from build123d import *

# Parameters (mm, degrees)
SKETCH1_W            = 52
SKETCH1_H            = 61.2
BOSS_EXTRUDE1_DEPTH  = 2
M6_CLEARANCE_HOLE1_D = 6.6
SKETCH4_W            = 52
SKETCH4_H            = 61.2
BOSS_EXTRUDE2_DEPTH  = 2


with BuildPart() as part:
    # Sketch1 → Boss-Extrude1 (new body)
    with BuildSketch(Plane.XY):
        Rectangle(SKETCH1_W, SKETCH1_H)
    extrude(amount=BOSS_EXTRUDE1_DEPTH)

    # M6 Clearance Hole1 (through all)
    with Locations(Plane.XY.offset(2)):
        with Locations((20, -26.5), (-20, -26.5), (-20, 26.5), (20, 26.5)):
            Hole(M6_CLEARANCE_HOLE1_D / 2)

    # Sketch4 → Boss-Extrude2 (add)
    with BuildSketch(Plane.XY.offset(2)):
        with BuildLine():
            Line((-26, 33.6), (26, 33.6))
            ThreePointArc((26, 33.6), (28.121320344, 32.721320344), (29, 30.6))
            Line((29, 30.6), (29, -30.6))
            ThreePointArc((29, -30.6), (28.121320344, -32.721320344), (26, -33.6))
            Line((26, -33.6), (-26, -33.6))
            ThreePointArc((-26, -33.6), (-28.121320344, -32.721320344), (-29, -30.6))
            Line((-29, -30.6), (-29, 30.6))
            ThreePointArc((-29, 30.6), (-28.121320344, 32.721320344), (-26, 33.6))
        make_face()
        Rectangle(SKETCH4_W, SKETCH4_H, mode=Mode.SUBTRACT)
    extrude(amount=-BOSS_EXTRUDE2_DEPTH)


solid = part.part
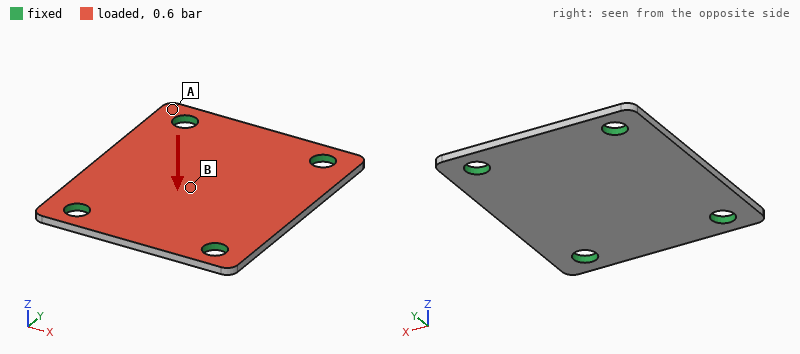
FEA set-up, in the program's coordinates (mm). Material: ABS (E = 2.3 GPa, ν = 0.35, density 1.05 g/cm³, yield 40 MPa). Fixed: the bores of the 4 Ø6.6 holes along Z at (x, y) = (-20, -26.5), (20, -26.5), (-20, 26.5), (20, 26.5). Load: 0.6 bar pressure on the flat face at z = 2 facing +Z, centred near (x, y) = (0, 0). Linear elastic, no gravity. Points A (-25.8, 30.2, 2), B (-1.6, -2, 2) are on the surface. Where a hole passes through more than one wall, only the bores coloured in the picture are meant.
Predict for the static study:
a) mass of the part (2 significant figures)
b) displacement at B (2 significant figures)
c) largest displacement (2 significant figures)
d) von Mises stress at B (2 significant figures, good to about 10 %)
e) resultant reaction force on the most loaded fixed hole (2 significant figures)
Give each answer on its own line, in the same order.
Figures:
7.9 g
0.84 mm
0.85 mm
8.6 MPa
56 N
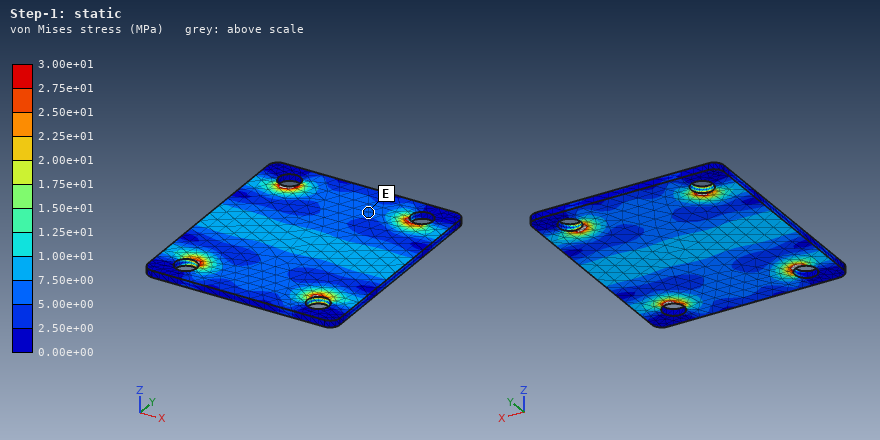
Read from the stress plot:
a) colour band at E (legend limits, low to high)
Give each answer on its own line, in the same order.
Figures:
5.00e+00 to 7.50e+00 MPa
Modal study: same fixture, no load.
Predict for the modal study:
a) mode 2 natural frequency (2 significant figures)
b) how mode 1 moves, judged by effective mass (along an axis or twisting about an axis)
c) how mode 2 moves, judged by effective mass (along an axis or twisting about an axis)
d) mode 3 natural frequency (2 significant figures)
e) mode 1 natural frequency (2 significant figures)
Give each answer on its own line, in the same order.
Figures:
1500 Hz
along Z
twisting about Y
1800 Hz
1100 Hz
